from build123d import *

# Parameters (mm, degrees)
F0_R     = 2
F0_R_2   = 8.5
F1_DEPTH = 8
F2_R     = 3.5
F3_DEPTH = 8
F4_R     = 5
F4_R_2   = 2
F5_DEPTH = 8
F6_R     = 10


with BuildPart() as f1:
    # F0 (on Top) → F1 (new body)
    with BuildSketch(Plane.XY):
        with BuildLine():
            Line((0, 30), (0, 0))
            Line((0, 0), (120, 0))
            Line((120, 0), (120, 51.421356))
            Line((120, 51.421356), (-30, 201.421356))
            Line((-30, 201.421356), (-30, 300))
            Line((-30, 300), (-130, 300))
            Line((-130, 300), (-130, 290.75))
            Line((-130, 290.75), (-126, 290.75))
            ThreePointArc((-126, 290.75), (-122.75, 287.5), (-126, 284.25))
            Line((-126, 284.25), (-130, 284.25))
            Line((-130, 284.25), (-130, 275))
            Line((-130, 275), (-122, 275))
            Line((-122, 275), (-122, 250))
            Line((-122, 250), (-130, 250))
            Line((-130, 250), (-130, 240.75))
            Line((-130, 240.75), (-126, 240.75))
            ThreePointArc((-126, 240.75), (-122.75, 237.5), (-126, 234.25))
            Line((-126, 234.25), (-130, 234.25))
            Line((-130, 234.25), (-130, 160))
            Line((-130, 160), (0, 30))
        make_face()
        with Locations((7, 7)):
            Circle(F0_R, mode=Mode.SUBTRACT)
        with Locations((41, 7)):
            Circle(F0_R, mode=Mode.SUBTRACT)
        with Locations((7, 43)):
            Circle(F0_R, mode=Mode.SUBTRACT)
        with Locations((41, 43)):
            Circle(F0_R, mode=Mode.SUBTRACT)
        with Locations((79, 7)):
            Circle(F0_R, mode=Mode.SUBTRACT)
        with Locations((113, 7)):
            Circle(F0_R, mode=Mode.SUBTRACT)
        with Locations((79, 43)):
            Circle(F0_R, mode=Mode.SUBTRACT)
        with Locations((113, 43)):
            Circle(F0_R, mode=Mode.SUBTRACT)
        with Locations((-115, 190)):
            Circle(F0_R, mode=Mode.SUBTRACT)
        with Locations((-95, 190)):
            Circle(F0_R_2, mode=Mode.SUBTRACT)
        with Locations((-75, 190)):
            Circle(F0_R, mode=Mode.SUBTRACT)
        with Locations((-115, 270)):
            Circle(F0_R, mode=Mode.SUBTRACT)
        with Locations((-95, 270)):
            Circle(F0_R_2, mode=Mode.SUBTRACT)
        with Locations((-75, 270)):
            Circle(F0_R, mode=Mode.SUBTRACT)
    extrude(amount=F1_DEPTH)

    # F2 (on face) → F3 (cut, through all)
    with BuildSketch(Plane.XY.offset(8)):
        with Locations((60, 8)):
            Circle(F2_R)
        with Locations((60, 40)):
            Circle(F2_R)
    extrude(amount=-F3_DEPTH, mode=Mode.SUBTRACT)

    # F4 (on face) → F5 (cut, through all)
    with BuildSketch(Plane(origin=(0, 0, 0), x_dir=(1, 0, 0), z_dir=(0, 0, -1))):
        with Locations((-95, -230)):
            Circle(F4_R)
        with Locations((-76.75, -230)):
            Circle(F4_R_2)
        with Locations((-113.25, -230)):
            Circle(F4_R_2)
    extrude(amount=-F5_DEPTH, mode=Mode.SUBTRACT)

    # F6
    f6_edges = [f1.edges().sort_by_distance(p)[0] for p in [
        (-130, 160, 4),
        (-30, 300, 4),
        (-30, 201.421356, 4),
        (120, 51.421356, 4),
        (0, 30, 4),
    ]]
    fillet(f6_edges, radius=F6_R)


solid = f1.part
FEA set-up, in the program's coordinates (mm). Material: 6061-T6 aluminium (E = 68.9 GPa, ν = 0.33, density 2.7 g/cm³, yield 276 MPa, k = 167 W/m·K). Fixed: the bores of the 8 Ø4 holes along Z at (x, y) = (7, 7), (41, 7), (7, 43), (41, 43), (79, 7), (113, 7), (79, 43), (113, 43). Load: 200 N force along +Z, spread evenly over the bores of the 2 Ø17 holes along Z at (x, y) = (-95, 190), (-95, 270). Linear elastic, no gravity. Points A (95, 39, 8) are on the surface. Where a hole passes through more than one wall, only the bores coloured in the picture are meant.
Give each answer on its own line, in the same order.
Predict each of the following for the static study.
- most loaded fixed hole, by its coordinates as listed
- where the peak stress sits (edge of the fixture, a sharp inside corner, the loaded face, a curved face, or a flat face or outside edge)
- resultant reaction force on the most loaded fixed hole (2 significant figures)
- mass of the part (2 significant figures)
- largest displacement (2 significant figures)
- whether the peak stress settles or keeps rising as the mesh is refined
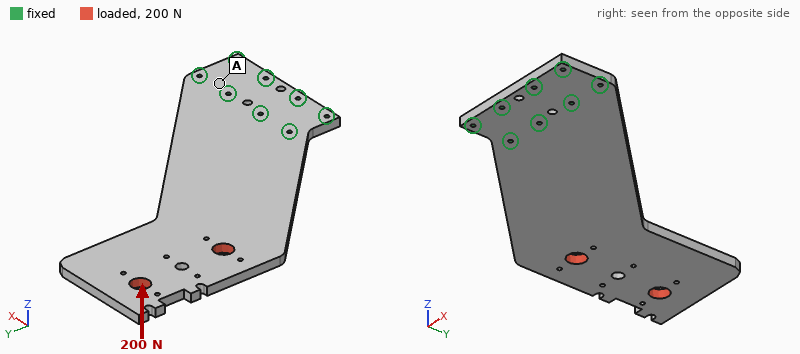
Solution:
(7, 43)
edge of the fixture
680 N
770 g
3.8 mm
keeps rising
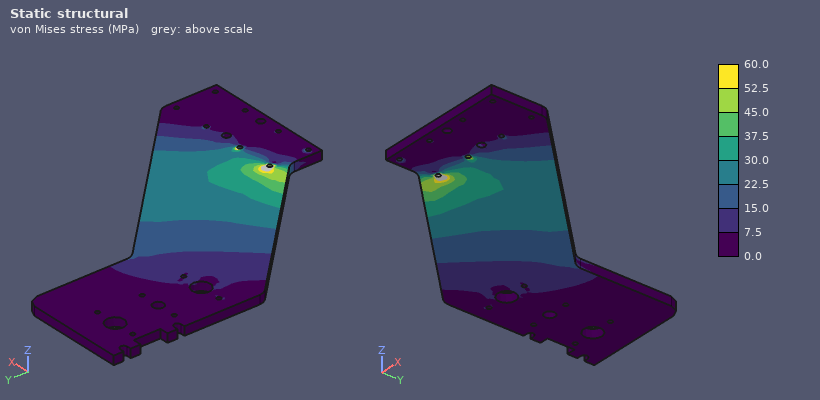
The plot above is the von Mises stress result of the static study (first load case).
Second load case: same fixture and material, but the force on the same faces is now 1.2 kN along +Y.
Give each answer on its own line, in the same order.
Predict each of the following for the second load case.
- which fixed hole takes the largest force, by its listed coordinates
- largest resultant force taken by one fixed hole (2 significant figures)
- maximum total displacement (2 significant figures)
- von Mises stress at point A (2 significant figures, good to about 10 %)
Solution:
(7, 43)
2.1 kN
0.11 mm
1.7 MPa
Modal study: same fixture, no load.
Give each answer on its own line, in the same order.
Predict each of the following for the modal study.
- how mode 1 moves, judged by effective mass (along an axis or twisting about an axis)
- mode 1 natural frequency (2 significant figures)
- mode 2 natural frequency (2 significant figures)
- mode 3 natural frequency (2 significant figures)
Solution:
along Z
84 Hz
370 Hz
550 Hz
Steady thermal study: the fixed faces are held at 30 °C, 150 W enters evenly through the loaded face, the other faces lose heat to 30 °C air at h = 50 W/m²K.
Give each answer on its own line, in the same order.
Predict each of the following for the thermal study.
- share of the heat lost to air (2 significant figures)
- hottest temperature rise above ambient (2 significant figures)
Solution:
83 %
84 K
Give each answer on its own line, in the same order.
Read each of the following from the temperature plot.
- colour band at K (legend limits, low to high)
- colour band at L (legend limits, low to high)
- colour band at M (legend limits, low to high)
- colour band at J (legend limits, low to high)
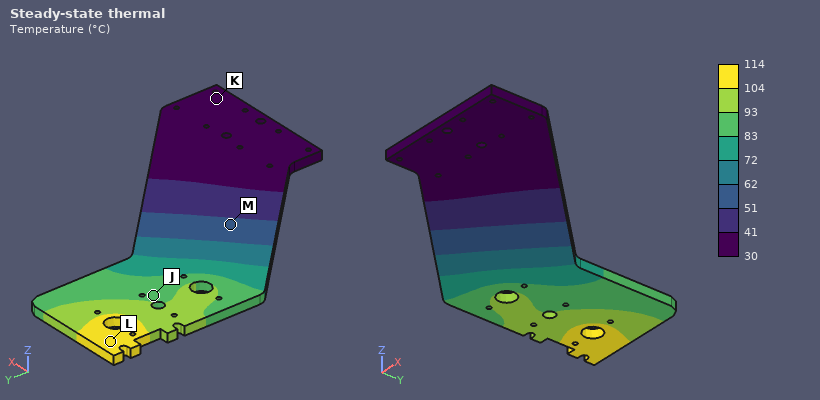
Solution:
30 to 41 °C
104 to 114 °C
51 to 62 °C
83 to 93 °C
